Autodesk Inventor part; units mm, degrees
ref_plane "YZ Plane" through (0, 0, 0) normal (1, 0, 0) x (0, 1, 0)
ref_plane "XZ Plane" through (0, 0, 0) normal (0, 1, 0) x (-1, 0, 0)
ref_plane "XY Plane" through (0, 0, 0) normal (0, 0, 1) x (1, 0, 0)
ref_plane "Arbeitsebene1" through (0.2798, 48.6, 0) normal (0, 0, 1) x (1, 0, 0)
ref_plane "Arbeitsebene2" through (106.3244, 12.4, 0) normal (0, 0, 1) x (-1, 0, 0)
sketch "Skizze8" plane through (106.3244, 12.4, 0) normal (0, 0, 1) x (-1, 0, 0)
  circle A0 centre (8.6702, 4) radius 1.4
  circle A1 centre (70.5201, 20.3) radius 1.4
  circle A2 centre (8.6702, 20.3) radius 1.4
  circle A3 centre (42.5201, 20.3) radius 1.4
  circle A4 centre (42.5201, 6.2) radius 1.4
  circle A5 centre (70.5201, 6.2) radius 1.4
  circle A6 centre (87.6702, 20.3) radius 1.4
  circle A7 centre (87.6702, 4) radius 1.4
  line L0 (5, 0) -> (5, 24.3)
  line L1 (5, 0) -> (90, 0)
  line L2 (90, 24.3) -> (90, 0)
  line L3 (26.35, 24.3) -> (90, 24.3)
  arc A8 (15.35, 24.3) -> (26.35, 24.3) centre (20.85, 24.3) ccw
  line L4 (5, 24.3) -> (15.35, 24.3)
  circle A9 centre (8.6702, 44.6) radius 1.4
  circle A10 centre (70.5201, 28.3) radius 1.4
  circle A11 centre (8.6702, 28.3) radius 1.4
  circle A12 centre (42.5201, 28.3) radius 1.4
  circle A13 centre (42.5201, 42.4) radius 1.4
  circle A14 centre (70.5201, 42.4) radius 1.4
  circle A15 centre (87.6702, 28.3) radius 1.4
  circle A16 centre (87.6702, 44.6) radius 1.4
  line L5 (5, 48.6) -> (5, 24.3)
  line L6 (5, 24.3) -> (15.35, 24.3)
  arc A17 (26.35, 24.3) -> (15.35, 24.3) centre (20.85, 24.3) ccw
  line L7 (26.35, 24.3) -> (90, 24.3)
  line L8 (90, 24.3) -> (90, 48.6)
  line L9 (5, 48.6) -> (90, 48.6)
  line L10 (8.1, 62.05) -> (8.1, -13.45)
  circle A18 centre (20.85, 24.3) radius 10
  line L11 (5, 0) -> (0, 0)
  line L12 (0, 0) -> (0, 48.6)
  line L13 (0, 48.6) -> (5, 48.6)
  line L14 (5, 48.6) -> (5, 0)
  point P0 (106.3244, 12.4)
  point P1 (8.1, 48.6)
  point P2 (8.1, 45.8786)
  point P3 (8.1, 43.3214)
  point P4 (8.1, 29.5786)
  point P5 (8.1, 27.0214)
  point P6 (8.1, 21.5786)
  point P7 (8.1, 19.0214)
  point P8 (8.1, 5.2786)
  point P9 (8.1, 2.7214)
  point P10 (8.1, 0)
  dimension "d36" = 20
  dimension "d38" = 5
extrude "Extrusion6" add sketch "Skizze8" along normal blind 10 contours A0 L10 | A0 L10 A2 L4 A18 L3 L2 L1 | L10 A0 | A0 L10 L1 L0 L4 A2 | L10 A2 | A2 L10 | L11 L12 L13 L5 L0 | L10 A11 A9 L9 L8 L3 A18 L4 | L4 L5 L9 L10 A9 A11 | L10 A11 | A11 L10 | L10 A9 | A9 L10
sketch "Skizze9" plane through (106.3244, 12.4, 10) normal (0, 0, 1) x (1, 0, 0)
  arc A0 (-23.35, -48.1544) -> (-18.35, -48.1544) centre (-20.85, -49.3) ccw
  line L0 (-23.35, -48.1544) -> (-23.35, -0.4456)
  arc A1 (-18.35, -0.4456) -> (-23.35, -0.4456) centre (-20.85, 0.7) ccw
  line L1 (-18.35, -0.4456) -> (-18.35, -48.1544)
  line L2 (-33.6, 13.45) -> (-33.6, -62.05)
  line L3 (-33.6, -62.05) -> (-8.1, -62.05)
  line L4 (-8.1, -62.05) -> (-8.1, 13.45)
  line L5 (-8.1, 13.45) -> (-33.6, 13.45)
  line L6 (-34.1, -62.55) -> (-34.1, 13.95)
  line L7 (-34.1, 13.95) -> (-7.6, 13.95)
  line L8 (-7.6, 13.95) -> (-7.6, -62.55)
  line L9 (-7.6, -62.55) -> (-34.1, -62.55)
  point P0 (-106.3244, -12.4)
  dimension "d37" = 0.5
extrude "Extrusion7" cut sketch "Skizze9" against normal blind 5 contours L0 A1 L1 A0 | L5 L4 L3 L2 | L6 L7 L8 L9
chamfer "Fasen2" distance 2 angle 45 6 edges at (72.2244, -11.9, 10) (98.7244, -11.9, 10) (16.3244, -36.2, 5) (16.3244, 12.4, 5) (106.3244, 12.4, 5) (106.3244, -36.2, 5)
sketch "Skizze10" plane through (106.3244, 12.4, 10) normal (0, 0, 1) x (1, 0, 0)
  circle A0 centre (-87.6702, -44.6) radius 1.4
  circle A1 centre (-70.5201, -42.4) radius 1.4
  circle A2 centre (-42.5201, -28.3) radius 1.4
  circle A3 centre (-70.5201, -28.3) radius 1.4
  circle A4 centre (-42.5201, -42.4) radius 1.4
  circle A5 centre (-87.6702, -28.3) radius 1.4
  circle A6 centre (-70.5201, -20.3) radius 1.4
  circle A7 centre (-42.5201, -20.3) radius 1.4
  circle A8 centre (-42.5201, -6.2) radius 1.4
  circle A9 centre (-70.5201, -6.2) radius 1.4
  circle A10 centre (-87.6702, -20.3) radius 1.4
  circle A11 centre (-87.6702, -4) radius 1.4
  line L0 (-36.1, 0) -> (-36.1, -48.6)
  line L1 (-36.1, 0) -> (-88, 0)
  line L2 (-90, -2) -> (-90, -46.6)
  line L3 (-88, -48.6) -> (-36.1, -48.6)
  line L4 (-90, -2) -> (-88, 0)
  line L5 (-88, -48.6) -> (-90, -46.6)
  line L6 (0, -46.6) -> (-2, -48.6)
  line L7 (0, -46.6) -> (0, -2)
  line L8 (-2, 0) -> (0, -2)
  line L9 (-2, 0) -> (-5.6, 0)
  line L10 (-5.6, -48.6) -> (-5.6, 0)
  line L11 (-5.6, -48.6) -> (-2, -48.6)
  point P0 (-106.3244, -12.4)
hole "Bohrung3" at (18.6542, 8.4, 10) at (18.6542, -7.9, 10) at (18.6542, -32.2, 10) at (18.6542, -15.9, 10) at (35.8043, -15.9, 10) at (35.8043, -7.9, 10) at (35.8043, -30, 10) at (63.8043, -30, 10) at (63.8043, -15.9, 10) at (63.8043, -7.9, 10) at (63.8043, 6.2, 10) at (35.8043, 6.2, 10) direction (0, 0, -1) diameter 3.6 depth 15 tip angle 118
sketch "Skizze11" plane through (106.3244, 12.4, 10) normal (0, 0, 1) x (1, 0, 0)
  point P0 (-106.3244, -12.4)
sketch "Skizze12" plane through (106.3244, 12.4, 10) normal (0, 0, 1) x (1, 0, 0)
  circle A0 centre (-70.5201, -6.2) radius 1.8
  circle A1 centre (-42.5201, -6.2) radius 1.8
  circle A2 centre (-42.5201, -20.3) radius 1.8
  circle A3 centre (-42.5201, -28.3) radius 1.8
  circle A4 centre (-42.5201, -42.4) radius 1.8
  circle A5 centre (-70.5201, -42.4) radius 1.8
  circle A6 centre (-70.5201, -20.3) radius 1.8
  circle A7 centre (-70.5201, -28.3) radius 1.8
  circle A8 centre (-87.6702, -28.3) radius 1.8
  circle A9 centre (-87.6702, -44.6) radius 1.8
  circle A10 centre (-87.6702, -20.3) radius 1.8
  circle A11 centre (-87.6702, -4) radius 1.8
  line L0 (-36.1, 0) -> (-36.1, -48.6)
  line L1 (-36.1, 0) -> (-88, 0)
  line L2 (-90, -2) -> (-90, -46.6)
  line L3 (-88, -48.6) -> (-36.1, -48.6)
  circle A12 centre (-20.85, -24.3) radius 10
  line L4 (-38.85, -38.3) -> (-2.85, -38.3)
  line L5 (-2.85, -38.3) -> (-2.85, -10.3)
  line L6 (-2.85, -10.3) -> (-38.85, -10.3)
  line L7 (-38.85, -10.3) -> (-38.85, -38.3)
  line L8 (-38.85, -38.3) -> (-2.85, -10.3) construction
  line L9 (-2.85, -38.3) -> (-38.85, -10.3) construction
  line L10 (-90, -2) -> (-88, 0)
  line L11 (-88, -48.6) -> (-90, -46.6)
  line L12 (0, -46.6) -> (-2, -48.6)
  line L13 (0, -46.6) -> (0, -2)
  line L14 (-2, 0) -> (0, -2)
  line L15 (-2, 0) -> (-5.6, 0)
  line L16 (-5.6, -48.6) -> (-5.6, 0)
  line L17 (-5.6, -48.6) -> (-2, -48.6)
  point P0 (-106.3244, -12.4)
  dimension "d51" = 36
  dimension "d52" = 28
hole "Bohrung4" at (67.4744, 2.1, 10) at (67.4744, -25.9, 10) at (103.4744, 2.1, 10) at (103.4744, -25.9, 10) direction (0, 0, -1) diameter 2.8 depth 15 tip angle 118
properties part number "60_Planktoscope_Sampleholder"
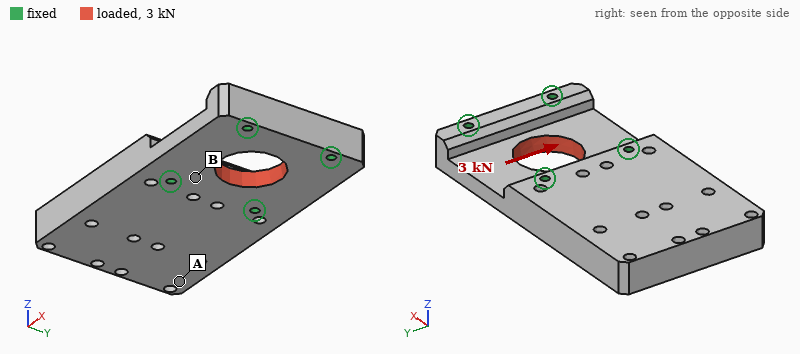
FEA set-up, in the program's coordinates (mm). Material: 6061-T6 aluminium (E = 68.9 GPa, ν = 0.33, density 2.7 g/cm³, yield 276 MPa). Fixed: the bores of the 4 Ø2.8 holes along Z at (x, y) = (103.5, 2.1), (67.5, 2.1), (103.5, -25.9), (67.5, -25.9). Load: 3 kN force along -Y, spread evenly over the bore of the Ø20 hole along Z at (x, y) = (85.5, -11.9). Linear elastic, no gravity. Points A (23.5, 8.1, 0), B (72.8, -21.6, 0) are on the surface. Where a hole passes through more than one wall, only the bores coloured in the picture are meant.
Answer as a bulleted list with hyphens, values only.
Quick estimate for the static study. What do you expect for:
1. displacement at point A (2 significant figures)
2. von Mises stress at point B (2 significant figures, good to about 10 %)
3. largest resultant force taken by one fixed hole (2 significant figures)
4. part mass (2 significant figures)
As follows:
- 0.85 µm
- 11 MPa
- 820 N
- 92 g
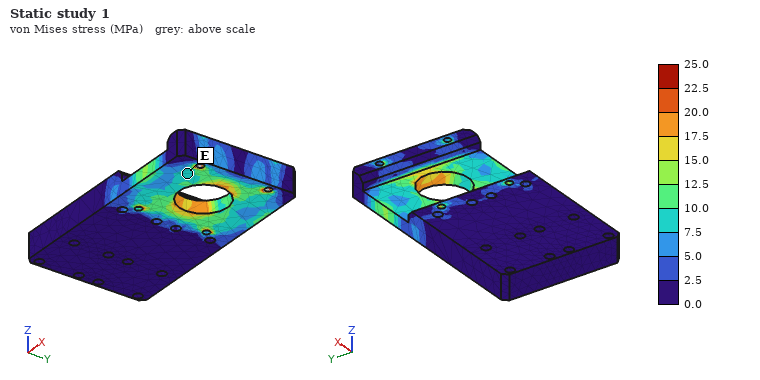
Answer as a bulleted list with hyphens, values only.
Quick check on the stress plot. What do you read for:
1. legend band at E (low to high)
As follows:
- 7.5 to 10.0 MPa
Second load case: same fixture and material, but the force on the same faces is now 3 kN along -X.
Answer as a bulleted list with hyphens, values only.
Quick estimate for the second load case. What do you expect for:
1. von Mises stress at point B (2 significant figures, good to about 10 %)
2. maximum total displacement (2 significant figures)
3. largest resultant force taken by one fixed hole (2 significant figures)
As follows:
- 11 MPa
- 4.8 µm
- 790 N
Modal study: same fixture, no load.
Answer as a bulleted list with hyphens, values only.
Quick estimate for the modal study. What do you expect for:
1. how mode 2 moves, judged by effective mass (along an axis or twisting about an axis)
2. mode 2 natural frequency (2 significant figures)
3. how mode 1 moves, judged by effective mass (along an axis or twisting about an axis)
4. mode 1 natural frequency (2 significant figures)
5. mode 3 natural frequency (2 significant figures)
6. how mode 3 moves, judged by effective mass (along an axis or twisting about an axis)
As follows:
- twisting about X
- 6500 Hz
- along Z
- 2600 Hz
- 8300 Hz
- along Y
